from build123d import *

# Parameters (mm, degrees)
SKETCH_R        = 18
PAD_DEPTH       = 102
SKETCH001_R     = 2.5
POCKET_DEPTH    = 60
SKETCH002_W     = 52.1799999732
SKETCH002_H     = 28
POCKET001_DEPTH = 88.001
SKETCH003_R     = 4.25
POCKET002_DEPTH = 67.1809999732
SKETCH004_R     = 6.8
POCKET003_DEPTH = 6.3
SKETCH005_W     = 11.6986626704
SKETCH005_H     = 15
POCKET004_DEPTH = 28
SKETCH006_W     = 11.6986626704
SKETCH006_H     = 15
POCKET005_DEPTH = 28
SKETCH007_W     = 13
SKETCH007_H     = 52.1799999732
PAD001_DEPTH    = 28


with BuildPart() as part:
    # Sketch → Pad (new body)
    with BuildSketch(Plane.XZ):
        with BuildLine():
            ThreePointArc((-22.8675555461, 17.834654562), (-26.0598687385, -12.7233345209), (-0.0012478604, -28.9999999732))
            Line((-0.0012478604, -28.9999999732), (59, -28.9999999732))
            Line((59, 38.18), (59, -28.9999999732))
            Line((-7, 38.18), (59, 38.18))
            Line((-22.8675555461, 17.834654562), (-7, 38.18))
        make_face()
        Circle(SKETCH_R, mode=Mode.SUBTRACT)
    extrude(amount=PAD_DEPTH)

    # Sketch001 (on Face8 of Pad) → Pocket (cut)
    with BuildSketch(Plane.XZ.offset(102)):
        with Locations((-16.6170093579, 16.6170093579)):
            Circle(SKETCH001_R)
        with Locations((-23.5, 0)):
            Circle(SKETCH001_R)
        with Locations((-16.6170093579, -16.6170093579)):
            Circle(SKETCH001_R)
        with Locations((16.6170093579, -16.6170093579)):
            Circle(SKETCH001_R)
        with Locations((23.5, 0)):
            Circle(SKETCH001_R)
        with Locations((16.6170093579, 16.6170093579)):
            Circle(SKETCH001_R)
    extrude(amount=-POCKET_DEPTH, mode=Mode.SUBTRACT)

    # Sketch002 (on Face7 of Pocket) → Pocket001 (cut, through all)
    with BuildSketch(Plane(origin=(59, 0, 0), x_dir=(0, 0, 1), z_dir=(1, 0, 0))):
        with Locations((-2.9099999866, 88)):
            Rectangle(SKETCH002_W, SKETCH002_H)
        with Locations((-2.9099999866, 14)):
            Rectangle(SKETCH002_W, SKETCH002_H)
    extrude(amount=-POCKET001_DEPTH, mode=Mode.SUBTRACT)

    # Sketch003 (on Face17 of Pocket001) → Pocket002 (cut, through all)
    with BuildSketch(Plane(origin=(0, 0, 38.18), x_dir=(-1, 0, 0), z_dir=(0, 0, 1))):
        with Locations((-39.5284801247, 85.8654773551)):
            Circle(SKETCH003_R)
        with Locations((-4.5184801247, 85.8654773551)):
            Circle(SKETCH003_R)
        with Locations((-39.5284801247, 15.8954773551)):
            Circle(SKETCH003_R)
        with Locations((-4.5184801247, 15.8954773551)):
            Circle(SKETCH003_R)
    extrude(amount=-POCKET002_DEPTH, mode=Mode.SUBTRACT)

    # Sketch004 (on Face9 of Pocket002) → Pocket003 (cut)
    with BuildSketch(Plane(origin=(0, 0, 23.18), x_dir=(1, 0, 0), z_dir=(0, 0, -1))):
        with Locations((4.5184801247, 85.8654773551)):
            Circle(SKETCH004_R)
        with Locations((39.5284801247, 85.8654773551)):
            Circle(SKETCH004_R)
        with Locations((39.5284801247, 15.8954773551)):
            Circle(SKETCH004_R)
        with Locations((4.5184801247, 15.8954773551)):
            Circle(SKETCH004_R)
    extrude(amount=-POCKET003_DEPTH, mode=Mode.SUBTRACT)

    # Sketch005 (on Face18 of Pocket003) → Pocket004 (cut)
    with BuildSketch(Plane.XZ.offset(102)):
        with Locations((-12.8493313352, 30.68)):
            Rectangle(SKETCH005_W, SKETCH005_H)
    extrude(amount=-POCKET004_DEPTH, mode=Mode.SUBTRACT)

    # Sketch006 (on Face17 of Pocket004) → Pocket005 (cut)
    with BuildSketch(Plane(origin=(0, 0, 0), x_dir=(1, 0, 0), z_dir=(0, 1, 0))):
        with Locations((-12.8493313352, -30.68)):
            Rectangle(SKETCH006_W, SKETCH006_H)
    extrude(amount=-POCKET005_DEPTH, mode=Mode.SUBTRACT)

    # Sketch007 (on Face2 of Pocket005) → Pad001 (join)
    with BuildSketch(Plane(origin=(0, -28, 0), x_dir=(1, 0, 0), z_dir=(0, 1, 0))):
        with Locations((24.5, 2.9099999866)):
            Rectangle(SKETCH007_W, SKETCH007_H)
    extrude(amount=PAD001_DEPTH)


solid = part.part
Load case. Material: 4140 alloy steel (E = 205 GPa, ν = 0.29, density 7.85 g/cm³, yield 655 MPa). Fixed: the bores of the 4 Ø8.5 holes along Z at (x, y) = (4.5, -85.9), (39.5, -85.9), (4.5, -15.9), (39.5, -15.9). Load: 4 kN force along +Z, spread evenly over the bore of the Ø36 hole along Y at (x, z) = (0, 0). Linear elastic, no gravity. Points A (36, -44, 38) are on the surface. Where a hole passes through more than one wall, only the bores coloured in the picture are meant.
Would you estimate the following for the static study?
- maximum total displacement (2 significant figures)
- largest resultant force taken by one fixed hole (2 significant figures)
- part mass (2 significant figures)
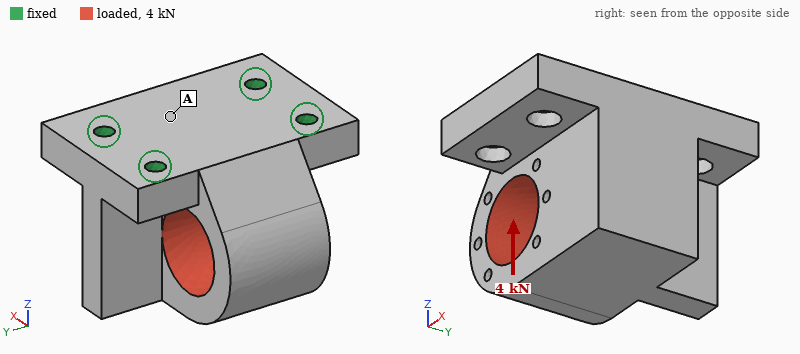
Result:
7.3 µm
2.5 kN
2.1 kg
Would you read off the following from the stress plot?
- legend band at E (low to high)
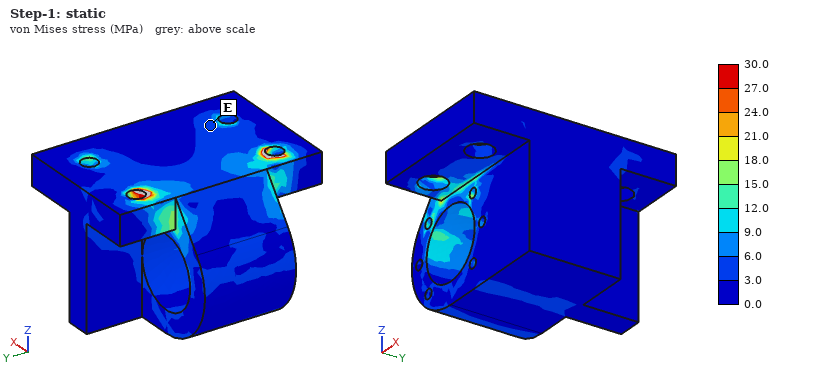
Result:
3.0 to 6.0 MPa
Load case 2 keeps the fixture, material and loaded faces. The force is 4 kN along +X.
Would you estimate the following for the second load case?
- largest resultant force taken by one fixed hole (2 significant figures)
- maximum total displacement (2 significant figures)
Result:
2.4 kN
8.6 µm
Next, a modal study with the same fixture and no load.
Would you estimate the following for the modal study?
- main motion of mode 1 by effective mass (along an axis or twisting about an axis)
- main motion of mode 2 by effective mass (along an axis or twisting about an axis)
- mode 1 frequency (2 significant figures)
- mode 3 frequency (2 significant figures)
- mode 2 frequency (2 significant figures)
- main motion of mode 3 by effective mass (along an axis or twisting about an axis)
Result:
along X
along Y
3200 Hz
7400 Hz
5500 Hz
along Z
